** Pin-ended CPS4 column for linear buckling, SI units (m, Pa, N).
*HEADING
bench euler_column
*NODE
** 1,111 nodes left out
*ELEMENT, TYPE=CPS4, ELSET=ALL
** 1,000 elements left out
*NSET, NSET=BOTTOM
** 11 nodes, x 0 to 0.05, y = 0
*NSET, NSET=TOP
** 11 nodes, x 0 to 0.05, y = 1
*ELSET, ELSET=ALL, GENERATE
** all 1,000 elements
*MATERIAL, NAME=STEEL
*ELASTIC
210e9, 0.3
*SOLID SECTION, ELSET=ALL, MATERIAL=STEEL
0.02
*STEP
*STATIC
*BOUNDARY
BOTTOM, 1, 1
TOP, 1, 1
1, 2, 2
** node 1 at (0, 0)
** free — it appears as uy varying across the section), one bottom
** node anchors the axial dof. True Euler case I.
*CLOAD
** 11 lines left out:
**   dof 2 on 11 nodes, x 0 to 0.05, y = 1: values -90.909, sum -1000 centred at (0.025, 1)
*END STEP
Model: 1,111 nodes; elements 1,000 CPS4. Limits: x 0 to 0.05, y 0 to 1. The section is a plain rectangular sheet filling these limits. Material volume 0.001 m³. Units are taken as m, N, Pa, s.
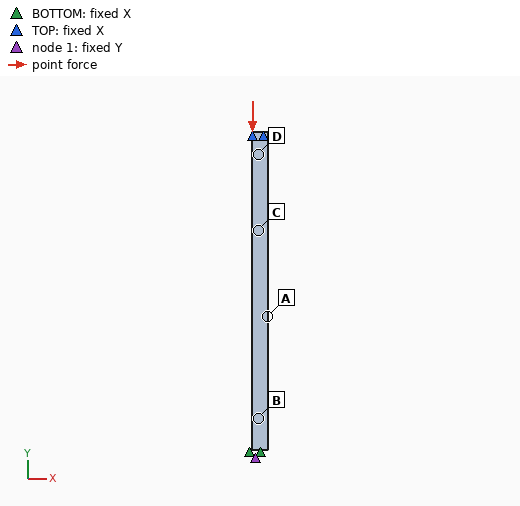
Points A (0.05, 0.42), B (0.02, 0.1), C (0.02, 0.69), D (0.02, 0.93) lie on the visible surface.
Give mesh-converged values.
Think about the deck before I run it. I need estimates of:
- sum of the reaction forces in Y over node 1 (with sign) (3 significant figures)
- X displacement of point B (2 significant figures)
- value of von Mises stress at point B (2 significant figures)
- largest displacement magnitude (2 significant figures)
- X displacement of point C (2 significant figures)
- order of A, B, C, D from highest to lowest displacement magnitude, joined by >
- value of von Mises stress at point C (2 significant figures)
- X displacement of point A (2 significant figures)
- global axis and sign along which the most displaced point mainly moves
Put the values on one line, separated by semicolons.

1000 N; 1.6e-05 m; 1.5e+06 Pa; 3.7e-05 m; 2.7e-05 m; A > C > B > D; 1.2e+06 Pa; 3.7e-05 m; +X
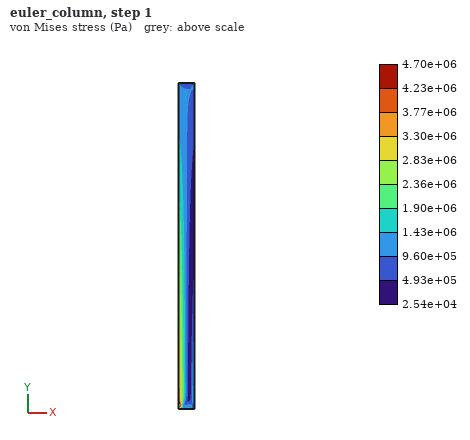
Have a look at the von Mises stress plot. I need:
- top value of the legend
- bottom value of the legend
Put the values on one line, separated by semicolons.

4.70e+06 Pa; 2.54e+04 Pa
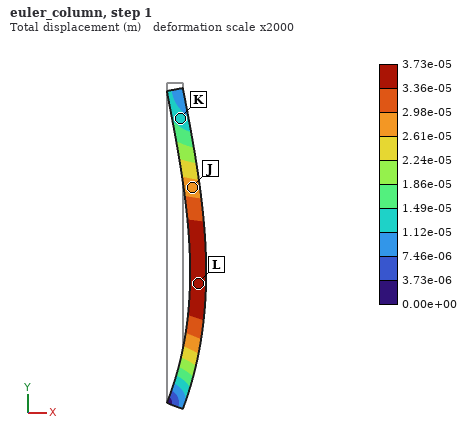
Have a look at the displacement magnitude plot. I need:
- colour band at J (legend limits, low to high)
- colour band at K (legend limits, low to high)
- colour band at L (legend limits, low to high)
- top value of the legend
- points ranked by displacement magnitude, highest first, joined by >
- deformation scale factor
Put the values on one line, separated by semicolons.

2.61e-05 to 2.98e-05 m; 1.12e-05 to 1.49e-05 m; 3.36e-05 to 3.73e-05 m; 3.73e-05 m; L > J > K; 2000
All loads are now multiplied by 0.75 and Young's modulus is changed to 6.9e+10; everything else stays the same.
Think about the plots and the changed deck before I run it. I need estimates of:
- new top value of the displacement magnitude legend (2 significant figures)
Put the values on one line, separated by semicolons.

8.5e-05 m
